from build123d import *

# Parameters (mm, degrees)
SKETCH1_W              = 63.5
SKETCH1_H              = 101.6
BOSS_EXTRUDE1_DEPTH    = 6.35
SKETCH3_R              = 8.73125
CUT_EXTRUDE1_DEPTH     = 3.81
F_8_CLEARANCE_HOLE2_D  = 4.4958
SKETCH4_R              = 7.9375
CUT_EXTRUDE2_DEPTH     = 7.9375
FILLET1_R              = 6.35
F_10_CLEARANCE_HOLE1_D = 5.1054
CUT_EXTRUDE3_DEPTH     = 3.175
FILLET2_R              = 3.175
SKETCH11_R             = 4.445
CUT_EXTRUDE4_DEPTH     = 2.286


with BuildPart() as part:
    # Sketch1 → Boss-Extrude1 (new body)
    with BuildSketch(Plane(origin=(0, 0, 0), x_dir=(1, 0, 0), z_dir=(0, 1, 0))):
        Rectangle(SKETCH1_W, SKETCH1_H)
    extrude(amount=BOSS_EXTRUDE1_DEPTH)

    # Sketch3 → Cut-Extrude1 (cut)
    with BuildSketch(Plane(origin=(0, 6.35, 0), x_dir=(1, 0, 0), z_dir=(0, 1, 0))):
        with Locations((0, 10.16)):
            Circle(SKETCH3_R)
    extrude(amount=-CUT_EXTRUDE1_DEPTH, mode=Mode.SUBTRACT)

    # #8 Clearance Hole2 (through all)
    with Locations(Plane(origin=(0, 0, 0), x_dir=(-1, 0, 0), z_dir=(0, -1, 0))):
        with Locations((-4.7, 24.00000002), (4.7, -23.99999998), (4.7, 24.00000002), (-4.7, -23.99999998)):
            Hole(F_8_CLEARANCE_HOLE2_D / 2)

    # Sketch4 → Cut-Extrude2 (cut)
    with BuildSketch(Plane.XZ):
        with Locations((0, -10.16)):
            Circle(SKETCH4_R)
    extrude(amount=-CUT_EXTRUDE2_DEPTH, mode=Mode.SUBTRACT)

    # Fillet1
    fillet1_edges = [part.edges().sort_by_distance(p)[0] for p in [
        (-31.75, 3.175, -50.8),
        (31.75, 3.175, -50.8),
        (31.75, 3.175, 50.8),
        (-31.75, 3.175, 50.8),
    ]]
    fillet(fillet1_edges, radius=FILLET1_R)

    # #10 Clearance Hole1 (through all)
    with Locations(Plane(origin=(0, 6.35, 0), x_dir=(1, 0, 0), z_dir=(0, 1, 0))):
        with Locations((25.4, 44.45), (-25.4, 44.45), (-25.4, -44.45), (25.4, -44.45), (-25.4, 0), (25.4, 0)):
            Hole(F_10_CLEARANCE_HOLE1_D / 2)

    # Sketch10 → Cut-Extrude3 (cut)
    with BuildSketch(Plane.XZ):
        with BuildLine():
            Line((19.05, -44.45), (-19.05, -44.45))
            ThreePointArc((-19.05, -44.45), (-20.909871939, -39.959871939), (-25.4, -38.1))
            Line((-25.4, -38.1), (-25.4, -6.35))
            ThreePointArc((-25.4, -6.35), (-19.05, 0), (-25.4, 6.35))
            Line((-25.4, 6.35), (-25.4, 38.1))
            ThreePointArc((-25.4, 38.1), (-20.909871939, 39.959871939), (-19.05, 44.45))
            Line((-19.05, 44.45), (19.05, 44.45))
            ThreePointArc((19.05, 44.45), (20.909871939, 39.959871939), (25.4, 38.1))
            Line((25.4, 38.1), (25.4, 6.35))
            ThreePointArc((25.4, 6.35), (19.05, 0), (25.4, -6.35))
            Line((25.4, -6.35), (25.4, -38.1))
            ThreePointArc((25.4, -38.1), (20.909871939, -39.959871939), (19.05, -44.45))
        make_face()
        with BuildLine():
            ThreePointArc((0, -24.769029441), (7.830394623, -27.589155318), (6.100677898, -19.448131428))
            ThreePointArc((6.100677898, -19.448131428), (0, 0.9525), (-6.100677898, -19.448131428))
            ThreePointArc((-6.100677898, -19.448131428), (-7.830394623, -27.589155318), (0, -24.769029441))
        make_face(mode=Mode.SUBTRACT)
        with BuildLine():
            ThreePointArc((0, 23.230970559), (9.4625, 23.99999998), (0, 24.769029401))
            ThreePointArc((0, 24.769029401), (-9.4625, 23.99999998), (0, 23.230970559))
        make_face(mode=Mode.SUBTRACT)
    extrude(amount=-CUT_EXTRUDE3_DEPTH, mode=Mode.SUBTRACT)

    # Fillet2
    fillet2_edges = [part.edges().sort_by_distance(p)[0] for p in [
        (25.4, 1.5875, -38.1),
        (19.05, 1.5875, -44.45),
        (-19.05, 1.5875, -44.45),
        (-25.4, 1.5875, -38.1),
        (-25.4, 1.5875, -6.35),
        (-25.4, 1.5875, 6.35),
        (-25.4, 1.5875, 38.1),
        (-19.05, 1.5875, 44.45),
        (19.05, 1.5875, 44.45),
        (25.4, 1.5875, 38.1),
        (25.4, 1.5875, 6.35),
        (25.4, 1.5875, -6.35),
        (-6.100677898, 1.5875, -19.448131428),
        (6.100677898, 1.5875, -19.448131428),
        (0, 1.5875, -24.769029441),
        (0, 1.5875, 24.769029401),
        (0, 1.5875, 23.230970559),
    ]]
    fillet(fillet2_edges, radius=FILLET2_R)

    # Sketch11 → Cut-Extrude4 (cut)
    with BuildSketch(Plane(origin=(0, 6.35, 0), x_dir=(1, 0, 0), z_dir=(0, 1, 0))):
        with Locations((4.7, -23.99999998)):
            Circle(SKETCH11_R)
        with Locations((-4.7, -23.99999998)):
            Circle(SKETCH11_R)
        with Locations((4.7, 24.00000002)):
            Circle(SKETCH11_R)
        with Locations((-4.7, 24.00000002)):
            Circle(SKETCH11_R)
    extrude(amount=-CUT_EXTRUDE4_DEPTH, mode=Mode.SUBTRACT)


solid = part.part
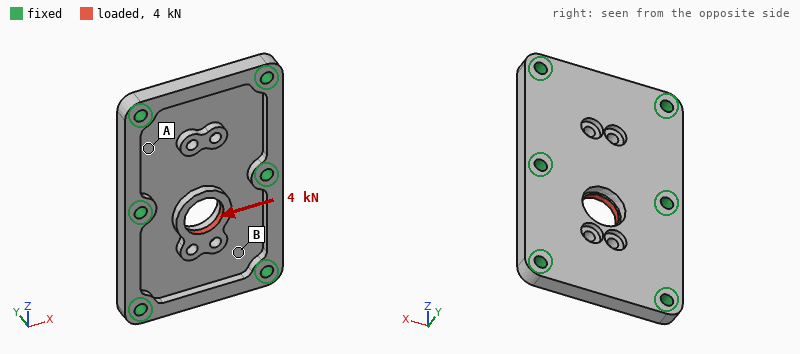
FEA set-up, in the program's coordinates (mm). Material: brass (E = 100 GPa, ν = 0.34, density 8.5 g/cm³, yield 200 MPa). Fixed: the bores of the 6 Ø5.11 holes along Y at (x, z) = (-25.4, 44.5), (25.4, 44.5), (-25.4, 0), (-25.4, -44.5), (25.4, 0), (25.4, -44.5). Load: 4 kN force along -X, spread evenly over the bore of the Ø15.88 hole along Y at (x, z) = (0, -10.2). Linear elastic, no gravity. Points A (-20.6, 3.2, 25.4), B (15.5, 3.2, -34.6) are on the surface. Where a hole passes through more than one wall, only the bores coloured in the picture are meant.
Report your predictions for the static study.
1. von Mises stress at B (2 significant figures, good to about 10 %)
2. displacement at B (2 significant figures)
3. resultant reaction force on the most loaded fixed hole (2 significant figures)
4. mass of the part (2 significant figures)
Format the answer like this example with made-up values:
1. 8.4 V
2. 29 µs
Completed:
1. 13 MPa
2. 4.3 µm
3. 1.4 kN
4. 220 g
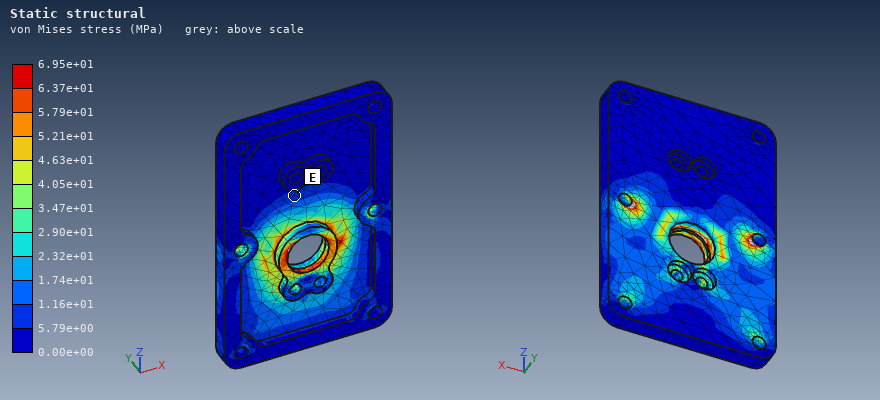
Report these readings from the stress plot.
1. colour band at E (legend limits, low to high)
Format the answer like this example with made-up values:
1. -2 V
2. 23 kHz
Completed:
1. 5.79e+00 to 1.16e+01 MPa
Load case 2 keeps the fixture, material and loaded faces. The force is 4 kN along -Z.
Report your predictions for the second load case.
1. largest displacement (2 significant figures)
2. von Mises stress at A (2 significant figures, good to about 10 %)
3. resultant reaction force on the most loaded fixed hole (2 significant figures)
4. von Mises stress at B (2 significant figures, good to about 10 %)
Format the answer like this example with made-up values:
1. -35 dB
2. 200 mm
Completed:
1. 23 µm
2. 5.4 MPa
3. 1.0 kN
4. 14 MPa
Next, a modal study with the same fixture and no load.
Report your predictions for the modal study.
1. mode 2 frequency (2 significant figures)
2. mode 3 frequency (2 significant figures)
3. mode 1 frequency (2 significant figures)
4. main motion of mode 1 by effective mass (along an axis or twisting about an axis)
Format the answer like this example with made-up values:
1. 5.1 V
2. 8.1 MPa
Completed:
1. 5400 Hz
2. 8000 Hz
3. 4900 Hz
4. along Y
